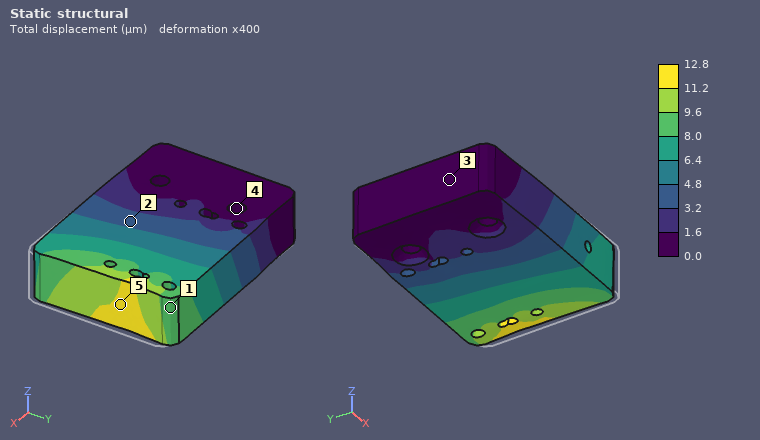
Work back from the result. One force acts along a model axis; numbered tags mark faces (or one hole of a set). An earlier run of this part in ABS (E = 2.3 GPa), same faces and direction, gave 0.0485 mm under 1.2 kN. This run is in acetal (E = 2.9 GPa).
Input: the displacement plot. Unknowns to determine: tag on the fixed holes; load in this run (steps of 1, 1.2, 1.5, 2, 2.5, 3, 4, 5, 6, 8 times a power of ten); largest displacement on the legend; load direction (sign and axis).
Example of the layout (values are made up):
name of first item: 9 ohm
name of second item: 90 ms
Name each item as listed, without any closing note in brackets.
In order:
tag on the fixed holes: 4
load in this run: 400 N
largest displacement on the legend: 12.8 µm
load direction: -X
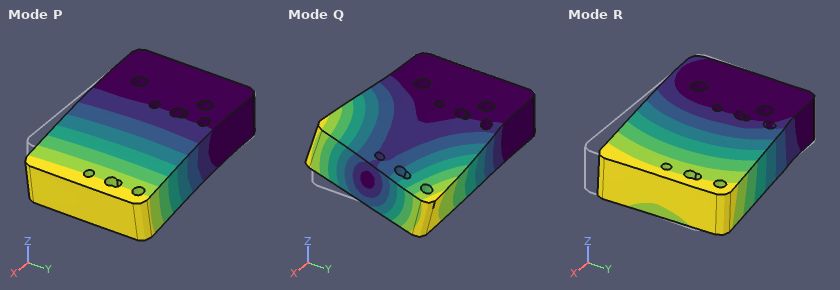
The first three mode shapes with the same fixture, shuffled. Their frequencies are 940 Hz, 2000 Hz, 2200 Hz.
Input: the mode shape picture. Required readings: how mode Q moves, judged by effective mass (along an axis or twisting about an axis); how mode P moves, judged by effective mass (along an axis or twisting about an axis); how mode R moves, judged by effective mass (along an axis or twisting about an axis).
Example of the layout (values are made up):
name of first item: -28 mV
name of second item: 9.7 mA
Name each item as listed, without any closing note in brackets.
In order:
how mode Q moves, judged by effective mass: twisting about X
how mode P moves, judged by effective mass: along Z
how mode R moves, judged by effective mass: along Y
